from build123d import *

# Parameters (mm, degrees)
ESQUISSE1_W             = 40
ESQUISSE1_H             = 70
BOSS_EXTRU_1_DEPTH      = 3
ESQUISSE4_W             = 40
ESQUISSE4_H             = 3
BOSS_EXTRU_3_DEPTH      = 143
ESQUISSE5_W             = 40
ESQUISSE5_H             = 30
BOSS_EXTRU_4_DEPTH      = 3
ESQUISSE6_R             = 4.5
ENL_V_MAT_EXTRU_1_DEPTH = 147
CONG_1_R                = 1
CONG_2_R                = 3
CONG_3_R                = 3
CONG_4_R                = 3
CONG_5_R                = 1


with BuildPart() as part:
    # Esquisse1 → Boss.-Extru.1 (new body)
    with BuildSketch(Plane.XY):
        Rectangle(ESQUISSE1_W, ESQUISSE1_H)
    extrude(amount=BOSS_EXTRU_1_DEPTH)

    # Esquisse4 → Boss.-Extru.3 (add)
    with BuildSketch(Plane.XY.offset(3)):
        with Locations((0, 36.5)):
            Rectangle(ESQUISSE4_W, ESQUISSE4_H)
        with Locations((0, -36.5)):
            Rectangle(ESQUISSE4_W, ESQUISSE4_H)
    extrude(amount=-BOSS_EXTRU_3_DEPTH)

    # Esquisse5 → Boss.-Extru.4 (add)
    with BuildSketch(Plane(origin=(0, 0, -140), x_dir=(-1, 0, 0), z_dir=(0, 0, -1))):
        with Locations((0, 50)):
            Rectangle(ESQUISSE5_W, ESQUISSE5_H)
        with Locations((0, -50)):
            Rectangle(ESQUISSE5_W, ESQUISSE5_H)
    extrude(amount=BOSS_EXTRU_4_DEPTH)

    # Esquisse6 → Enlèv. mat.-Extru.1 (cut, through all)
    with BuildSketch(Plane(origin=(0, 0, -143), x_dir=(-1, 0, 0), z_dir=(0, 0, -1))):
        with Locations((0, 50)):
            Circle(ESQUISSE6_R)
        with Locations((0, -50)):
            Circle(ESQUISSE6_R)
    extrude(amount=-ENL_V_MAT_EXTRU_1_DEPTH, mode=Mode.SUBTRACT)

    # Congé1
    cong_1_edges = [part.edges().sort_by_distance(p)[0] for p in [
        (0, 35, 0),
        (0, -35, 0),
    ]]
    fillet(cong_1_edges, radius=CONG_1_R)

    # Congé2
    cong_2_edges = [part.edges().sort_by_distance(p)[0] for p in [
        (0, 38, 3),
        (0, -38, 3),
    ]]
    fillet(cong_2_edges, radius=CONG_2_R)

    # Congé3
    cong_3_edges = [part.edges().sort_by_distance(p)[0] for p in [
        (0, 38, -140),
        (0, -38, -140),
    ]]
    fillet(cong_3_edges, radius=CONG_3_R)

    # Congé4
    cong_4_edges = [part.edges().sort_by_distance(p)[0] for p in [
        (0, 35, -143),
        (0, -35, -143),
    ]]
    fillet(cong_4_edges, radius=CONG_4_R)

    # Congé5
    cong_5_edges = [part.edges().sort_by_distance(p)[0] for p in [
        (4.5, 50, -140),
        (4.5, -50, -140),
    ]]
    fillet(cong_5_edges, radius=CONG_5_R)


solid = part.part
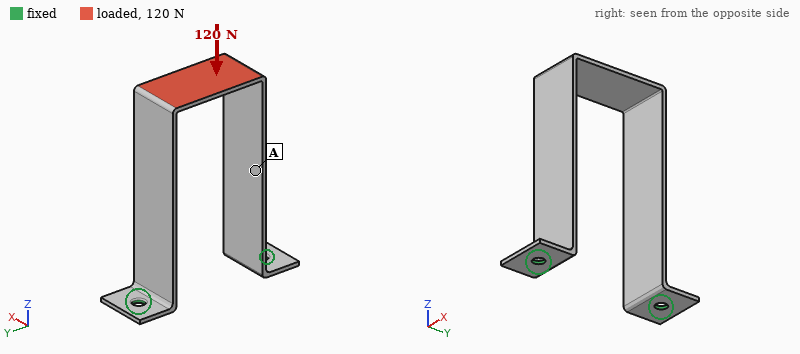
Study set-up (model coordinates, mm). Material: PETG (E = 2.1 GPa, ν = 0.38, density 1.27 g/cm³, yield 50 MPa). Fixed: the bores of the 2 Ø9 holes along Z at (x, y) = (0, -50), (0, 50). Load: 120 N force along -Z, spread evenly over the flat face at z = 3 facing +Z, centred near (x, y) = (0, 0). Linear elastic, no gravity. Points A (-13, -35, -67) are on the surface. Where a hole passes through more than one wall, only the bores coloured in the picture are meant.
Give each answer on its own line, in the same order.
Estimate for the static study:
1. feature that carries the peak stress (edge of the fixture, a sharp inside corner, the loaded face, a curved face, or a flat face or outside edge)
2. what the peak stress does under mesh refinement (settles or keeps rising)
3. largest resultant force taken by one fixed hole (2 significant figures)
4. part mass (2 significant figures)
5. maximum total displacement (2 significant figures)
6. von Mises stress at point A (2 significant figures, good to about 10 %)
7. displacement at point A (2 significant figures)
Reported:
edge of the fixture
keeps rising
60 N
63 g
2.1 mm
2.0 MPa
1.1 mm
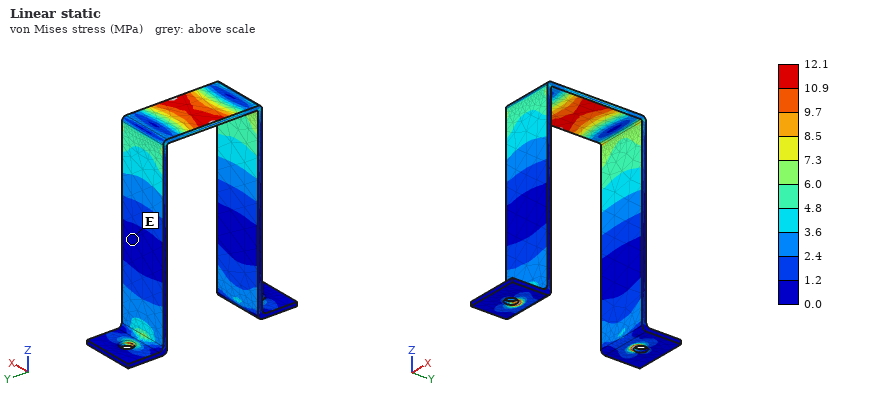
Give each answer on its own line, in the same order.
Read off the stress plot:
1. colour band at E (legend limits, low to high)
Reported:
0.0 to 1.2 MPa
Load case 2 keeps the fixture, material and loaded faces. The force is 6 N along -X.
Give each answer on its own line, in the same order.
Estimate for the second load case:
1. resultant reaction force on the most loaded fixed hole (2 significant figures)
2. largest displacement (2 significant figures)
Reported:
3.0 N
1.8 mm
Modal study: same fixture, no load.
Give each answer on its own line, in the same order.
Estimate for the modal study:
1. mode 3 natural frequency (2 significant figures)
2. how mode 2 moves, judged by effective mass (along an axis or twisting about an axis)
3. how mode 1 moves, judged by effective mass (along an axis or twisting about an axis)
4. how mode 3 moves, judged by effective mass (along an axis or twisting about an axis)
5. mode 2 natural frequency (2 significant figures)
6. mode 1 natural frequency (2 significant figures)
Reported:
90 Hz
along X
along Y
twisting about Z
58 Hz
34 Hz
